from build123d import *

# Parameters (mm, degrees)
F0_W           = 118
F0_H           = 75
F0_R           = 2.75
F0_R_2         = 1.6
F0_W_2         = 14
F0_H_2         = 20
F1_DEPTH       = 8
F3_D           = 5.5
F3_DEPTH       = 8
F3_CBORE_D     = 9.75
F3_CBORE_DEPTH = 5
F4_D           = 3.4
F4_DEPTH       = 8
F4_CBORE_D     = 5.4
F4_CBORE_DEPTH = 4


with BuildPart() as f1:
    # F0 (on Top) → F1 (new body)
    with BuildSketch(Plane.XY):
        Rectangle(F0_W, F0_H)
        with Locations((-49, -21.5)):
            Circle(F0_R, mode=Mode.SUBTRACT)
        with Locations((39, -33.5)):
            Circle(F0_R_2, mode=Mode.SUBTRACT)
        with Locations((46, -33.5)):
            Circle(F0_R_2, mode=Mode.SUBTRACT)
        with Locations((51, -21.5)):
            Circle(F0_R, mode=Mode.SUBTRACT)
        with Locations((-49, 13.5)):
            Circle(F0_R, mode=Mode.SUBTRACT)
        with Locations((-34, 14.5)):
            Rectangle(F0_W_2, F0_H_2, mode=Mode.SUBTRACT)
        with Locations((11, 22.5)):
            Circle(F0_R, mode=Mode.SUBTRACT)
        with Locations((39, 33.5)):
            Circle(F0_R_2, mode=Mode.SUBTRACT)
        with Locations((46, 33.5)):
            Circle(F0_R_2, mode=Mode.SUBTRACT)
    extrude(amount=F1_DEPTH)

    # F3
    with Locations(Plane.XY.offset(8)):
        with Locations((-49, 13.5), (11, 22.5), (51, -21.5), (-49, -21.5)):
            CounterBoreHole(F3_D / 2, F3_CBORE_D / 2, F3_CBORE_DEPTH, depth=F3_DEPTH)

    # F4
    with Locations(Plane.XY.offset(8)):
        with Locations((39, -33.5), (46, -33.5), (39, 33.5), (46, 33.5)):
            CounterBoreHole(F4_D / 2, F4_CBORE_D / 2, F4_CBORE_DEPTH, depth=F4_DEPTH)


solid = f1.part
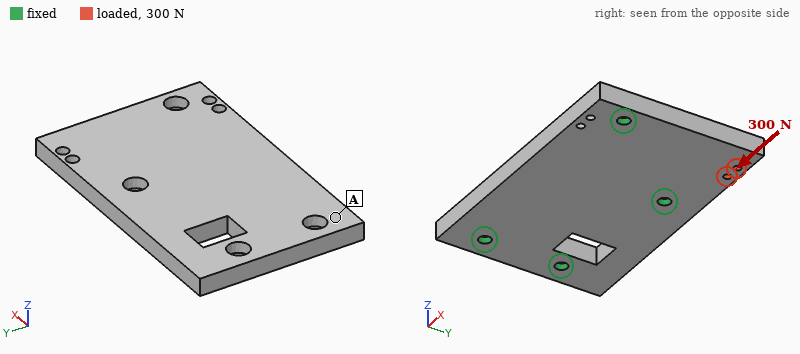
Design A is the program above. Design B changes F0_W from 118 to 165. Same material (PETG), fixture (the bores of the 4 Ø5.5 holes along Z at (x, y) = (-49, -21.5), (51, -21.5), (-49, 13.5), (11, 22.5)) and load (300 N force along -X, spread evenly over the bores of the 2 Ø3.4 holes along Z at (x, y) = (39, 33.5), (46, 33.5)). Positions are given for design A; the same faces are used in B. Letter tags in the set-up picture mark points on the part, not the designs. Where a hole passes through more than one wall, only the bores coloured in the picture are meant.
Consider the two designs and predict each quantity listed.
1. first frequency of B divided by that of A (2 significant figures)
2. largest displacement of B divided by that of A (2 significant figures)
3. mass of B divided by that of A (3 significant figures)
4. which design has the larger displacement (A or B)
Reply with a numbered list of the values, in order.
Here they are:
1. 0.60
2. 1.1
3. 1.43
4. B
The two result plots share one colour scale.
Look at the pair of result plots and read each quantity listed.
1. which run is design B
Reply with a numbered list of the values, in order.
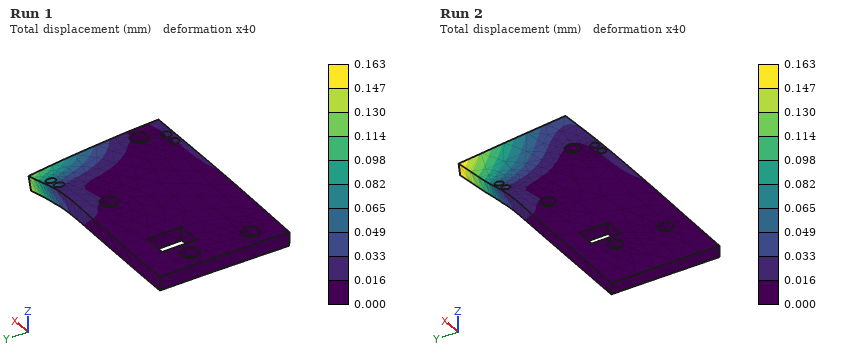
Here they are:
1. Run 2
